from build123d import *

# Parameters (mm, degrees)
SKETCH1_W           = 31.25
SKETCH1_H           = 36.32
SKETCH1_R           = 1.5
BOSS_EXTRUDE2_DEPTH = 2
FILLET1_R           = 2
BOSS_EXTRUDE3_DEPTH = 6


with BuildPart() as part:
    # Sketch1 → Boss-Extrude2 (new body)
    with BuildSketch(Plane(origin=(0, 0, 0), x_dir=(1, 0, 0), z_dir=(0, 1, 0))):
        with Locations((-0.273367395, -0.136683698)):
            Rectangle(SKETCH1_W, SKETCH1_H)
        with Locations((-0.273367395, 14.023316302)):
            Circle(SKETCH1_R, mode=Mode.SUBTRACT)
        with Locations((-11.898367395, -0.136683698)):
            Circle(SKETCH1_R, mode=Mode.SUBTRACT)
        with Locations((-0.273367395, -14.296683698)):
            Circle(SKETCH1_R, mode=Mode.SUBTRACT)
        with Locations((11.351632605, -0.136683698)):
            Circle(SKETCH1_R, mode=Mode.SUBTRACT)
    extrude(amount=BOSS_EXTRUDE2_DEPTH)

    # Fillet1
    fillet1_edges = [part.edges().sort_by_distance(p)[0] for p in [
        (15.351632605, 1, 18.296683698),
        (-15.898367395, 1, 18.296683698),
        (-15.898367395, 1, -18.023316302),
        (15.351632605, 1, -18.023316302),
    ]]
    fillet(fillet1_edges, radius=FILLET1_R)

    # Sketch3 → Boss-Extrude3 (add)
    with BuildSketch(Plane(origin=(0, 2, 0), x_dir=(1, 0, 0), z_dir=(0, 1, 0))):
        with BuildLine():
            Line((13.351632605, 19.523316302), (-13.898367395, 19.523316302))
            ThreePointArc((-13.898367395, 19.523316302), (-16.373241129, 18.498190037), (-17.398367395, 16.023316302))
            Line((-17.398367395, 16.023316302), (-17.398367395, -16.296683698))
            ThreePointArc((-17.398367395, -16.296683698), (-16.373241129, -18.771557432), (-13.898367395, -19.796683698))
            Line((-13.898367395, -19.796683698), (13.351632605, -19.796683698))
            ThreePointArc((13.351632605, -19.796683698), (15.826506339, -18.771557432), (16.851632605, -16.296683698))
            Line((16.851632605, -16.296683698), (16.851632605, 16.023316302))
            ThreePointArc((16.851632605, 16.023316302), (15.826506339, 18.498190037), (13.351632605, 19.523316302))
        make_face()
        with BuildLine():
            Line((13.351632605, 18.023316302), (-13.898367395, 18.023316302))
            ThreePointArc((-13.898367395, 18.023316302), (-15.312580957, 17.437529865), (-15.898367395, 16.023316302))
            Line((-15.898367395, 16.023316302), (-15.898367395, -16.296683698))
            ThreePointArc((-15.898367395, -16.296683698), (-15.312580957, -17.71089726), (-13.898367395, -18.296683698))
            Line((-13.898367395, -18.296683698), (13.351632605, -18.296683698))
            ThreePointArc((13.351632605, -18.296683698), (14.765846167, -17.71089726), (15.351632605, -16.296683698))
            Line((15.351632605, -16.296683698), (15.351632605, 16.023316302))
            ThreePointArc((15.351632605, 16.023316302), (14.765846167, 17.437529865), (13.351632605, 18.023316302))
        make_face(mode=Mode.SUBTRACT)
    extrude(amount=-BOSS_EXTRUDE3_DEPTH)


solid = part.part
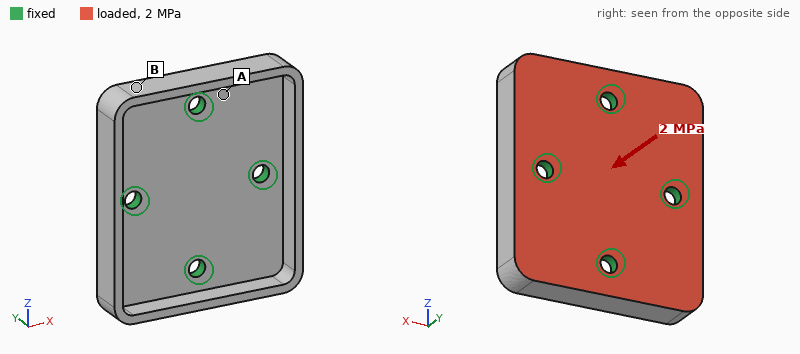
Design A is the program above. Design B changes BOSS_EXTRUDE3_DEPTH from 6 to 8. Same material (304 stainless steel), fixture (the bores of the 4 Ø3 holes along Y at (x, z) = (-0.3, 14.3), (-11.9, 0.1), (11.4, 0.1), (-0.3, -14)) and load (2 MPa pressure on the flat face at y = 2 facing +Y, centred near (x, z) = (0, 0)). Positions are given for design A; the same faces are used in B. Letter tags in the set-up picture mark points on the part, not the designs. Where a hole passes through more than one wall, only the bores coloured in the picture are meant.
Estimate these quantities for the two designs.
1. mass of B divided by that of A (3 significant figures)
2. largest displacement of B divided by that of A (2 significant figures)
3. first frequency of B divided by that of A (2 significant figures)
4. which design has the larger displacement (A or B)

1.12
0.64
0.88
A
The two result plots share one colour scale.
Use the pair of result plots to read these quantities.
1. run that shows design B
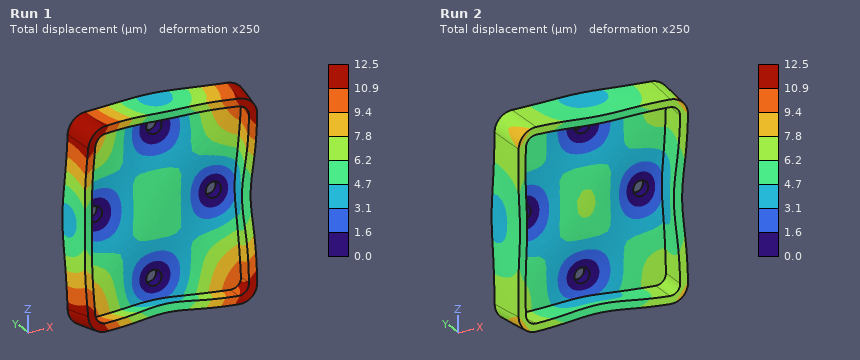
Run 2
